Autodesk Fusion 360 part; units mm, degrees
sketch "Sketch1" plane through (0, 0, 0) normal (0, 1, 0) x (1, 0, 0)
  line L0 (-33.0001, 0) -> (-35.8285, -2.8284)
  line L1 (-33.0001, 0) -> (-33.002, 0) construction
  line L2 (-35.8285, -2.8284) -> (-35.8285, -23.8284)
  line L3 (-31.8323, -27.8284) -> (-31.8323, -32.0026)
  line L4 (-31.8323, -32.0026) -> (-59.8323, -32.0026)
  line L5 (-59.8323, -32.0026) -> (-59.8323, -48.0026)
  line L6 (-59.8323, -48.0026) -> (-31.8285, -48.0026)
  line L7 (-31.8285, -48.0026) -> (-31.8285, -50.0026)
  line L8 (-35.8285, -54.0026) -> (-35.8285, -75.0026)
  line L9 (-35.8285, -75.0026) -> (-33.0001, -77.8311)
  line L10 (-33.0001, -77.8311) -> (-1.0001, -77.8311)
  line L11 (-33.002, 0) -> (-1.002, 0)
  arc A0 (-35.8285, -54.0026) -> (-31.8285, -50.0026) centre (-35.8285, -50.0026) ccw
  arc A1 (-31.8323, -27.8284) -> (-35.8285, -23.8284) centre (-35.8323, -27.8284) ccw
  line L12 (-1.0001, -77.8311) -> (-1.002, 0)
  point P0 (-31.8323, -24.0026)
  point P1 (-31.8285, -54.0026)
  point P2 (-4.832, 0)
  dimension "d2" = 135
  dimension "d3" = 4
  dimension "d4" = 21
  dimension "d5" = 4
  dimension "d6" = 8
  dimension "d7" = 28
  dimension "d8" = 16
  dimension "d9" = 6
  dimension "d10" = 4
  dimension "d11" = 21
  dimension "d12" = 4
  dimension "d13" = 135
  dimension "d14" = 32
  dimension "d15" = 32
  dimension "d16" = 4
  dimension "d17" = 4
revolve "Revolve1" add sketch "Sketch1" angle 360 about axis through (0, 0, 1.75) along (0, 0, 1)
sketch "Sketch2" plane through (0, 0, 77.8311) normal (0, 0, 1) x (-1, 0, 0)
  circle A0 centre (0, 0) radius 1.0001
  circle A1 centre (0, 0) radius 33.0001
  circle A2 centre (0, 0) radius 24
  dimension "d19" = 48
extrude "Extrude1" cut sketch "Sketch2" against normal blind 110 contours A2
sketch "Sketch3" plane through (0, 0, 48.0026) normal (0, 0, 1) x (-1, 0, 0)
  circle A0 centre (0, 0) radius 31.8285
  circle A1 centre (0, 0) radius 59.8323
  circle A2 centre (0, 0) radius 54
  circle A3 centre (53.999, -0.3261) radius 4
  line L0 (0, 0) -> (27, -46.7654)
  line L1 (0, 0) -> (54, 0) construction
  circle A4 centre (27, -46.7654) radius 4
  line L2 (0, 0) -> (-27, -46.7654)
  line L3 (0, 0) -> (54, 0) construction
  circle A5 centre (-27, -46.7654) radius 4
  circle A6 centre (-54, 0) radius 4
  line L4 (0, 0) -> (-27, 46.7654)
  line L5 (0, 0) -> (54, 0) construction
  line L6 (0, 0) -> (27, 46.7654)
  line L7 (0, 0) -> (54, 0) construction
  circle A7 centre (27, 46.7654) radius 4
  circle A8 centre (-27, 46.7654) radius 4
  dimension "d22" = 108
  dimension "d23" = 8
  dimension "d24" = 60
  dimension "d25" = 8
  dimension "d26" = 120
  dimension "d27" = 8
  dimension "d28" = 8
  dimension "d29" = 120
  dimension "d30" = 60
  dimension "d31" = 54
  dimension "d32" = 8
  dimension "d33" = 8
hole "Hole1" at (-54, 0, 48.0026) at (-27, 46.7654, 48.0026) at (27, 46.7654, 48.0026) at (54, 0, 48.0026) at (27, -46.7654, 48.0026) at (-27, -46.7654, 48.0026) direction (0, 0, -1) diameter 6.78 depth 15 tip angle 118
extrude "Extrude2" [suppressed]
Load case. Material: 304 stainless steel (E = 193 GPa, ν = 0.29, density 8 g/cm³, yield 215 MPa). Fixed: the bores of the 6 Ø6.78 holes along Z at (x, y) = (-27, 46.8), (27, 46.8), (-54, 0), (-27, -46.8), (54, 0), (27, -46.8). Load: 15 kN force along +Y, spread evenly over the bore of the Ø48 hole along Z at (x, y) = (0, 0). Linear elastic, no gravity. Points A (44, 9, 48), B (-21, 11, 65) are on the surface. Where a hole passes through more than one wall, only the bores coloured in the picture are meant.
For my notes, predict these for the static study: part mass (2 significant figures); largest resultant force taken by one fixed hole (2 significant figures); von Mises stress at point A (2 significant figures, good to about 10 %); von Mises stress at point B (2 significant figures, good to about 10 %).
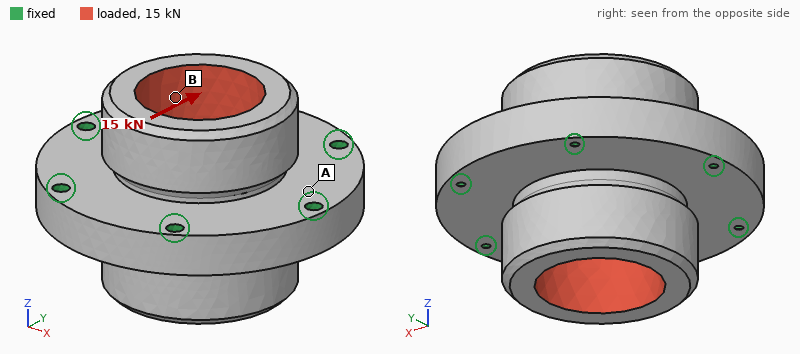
2.2 kg
3.0 kN
3.5 MPa
6.5 MPa
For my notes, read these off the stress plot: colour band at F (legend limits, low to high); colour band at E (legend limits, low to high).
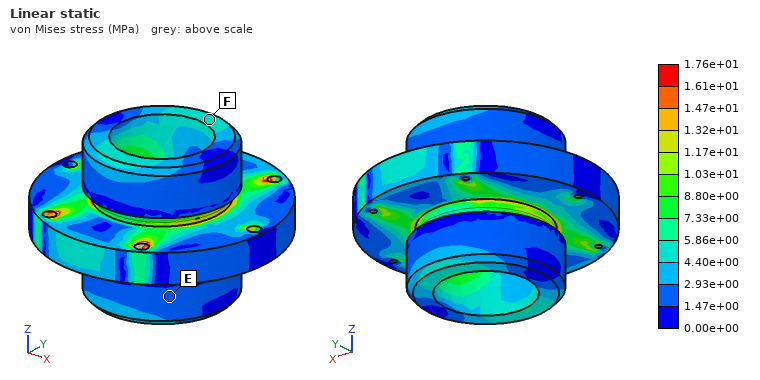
4.40e+00 to 5.86e+00 MPa
1.47e+00 to 2.93e+00 MPa
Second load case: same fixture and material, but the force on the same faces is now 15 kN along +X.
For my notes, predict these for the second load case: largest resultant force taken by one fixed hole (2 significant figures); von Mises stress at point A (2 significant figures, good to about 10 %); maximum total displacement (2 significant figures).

3.3 kN
6.6 MPa
4.1 µm
